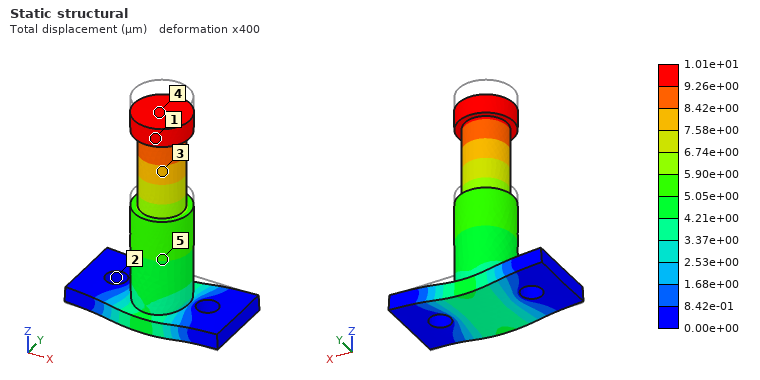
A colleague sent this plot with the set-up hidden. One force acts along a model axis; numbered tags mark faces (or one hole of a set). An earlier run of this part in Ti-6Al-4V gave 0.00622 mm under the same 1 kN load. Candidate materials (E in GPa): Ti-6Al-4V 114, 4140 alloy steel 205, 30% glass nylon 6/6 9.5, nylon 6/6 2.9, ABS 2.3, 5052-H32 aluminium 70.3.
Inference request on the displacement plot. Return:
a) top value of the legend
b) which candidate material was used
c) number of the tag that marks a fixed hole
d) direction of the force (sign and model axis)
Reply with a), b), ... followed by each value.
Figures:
a) 1.01e+01 µm
b) 5052-H32 aluminium
c) 2
d) -Z
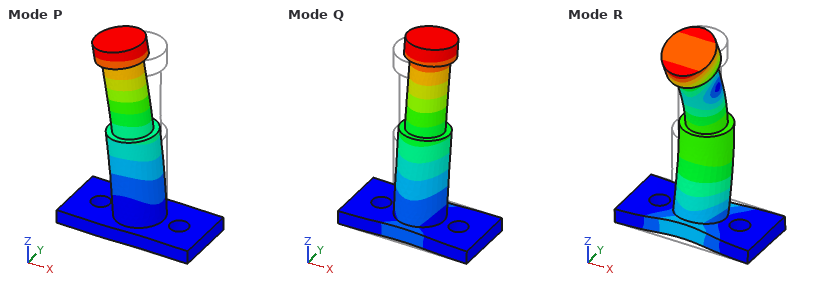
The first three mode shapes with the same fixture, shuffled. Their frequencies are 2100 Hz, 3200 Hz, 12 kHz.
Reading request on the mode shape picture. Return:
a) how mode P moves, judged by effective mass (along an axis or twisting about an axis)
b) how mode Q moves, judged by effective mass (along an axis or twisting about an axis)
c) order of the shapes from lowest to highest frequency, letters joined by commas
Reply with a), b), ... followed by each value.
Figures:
a) along X
b) along Y
c) Q, P, R
